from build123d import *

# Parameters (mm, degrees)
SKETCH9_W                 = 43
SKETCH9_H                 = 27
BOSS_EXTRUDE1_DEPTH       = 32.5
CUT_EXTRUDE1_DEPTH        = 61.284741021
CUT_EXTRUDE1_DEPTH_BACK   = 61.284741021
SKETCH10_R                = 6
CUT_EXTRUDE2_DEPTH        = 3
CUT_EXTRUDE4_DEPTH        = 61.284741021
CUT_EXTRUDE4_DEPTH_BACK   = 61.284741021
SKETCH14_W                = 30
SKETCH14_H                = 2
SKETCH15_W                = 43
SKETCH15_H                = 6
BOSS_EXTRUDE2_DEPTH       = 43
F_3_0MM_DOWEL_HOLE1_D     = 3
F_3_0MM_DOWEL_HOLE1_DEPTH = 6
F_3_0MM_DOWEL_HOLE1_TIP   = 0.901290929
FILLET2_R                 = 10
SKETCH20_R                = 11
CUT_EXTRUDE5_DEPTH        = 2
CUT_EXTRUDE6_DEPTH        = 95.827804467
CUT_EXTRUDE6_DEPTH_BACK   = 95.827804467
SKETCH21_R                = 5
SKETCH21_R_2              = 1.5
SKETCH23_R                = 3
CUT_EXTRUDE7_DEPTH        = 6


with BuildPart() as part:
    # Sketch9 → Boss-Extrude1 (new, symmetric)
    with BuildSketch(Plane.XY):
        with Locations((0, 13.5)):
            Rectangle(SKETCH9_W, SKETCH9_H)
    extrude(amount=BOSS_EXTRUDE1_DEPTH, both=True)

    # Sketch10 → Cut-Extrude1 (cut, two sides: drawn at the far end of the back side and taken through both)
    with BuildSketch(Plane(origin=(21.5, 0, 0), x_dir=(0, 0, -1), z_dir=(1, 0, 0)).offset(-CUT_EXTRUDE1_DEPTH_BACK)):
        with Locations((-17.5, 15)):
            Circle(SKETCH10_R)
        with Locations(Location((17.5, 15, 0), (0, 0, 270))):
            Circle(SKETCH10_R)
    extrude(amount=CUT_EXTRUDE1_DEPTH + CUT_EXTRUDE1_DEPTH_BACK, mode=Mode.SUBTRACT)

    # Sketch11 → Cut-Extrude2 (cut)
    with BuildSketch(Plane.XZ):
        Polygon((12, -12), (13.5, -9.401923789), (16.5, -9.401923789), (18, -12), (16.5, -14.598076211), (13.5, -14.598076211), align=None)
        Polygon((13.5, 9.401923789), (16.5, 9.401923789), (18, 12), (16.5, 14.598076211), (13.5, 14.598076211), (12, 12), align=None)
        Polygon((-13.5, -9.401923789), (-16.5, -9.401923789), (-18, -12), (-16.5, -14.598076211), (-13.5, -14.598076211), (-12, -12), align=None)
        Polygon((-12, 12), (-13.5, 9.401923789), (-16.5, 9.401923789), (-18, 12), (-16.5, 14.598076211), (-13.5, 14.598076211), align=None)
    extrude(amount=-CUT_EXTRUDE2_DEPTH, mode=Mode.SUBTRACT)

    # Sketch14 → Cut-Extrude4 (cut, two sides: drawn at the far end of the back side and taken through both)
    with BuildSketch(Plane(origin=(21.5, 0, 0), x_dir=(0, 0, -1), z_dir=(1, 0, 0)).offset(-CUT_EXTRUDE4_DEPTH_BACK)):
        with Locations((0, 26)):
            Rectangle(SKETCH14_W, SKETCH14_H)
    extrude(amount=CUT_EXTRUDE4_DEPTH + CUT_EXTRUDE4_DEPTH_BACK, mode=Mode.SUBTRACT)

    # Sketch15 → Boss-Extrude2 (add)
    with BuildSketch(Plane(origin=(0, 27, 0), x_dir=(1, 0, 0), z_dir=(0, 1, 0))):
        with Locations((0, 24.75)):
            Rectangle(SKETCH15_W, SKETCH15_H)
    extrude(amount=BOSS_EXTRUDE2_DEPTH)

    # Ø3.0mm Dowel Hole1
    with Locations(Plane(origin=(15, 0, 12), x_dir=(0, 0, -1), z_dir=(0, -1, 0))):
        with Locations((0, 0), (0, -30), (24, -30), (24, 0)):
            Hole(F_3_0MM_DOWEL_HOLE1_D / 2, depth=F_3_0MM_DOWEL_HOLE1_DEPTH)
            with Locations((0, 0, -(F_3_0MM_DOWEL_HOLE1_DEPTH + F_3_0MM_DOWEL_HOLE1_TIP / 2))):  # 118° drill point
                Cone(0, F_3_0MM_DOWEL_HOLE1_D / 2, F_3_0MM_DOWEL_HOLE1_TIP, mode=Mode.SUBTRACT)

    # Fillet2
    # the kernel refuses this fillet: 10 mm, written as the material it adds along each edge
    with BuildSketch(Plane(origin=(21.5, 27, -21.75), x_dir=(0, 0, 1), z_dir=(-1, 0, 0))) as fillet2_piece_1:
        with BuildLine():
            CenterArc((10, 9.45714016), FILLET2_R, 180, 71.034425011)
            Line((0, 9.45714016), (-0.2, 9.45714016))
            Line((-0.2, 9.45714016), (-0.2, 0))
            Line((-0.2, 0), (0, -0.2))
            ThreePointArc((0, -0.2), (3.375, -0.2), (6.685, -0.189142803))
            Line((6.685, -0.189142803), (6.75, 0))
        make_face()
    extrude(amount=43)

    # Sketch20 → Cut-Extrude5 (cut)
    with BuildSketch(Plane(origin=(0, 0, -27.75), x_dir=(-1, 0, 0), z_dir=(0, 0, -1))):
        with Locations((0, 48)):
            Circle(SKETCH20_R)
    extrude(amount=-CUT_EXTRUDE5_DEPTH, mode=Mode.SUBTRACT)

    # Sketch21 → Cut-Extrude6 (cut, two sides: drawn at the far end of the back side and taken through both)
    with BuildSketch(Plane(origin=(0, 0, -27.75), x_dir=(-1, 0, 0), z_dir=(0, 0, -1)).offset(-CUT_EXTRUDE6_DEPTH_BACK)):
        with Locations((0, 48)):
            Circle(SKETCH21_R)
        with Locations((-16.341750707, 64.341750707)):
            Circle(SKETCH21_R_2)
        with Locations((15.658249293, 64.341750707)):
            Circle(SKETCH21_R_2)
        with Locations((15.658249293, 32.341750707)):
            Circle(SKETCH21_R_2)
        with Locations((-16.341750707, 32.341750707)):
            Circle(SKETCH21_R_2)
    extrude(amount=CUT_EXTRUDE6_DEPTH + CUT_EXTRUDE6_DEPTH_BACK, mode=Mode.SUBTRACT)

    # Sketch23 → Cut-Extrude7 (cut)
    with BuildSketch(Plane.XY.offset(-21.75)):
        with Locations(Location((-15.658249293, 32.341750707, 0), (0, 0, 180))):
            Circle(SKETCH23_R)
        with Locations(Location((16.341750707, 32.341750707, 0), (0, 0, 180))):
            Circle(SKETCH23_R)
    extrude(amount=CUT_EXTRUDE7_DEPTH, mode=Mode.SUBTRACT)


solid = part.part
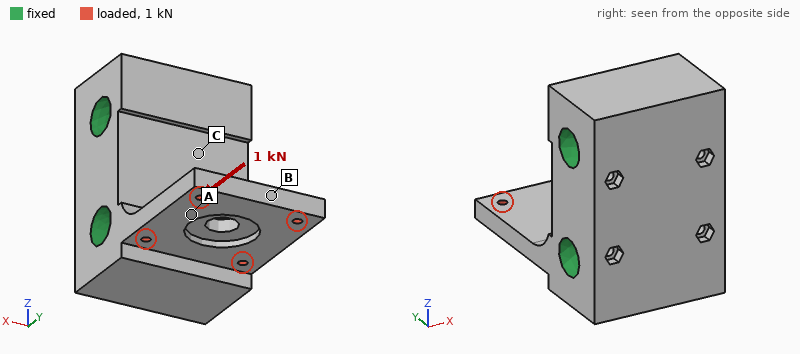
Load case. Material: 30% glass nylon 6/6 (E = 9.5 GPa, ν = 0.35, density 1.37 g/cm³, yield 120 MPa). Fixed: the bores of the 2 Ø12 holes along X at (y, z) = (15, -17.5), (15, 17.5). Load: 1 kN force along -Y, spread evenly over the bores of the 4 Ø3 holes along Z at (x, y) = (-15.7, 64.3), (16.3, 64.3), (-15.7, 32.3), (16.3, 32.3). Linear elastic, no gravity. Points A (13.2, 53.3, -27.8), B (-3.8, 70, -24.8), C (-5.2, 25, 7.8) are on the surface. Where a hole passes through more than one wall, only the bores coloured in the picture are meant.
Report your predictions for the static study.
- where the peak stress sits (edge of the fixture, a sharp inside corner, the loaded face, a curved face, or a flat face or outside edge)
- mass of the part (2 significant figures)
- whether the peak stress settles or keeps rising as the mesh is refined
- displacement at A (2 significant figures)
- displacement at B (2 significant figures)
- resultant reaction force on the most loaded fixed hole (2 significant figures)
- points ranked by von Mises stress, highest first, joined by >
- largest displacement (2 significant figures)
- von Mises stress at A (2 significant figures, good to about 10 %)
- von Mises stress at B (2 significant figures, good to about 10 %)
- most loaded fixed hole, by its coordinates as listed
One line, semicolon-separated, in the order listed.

a sharp inside corner; 100 g; keeps rising; 25 µm; 42 µm; 1.0 kN; A > B > C; 46 µm; 3.7 MPa; 1.7 MPa; (15, -17.5)
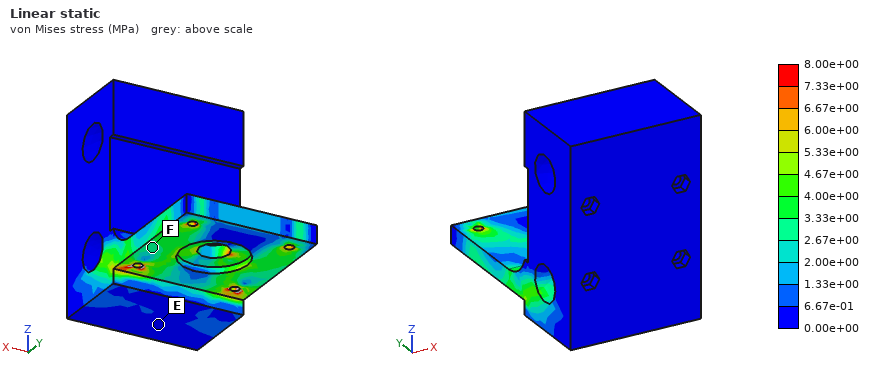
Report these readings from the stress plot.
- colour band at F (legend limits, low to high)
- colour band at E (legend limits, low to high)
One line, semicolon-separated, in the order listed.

2.67e+00 to 3.33e+00 MPa; 0.00e+00 to 6.67e-01 MPa
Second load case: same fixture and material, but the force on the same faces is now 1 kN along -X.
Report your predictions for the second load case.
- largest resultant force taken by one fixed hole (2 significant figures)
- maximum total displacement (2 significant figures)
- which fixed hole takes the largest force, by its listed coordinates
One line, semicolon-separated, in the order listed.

1.0 kN; 0.10 mm; (15, -17.5)
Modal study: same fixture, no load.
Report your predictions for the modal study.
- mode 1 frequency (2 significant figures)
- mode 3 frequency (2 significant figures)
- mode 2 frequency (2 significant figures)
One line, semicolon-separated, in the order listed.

1400 Hz; 5200 Hz; 2900 Hz
